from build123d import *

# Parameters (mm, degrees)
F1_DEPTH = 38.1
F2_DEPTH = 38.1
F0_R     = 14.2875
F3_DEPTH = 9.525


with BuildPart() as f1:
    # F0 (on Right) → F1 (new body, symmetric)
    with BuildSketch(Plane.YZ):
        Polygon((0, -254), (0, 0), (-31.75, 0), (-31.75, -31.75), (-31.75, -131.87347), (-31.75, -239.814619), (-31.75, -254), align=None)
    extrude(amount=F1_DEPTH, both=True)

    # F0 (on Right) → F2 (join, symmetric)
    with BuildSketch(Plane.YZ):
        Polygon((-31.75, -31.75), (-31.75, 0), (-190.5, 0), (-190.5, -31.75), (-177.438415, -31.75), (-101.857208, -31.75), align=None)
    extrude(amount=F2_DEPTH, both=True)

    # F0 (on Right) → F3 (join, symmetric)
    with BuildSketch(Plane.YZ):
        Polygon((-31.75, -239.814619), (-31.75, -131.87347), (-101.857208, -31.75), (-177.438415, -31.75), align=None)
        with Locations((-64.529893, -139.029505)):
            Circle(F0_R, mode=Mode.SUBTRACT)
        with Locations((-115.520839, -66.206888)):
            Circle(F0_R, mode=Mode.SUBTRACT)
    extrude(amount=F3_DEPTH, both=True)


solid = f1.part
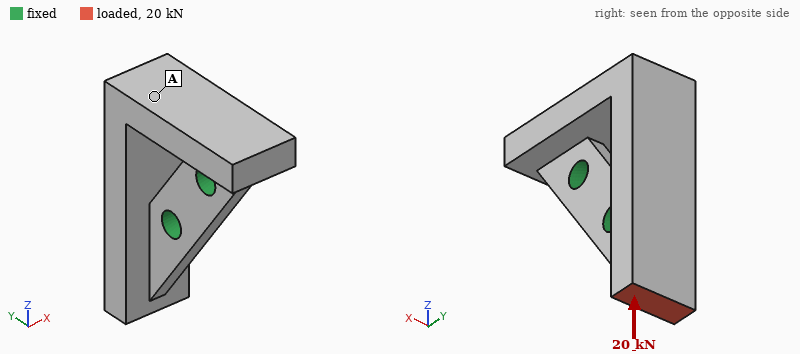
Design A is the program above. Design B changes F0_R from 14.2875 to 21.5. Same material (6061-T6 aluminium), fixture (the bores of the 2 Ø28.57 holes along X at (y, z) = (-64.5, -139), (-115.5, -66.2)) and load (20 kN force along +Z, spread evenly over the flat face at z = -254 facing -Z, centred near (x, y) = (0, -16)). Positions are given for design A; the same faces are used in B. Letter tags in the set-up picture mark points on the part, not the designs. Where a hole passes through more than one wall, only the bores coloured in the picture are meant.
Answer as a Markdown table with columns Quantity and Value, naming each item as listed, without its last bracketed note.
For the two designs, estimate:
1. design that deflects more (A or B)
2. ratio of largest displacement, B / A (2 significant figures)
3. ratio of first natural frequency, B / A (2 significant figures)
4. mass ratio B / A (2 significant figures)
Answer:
| Quantity | Value |
|---|---|
| design that deflects more | A |
| ratio of largest displacement, B / A | 0.70 |
| ratio of first natural frequency, B / A | 1.2 |
| mass ratio B / A | 0.97 |
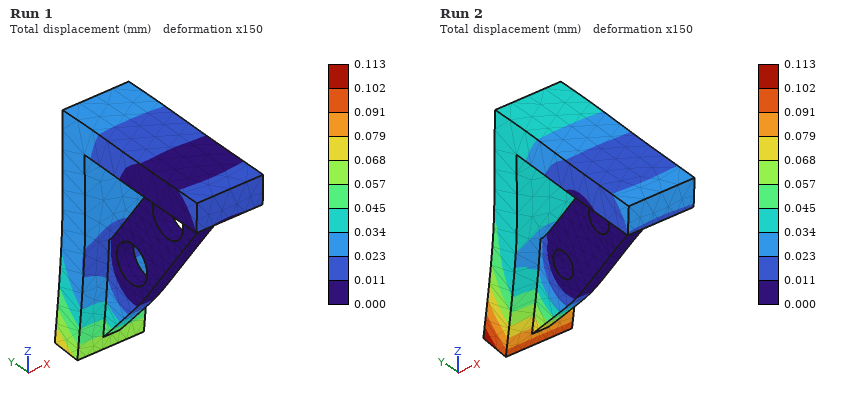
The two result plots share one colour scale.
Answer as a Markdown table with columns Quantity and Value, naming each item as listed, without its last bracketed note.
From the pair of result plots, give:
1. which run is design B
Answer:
| Quantity | Value |
|---|---|
| which run is design B | Run 1 |
